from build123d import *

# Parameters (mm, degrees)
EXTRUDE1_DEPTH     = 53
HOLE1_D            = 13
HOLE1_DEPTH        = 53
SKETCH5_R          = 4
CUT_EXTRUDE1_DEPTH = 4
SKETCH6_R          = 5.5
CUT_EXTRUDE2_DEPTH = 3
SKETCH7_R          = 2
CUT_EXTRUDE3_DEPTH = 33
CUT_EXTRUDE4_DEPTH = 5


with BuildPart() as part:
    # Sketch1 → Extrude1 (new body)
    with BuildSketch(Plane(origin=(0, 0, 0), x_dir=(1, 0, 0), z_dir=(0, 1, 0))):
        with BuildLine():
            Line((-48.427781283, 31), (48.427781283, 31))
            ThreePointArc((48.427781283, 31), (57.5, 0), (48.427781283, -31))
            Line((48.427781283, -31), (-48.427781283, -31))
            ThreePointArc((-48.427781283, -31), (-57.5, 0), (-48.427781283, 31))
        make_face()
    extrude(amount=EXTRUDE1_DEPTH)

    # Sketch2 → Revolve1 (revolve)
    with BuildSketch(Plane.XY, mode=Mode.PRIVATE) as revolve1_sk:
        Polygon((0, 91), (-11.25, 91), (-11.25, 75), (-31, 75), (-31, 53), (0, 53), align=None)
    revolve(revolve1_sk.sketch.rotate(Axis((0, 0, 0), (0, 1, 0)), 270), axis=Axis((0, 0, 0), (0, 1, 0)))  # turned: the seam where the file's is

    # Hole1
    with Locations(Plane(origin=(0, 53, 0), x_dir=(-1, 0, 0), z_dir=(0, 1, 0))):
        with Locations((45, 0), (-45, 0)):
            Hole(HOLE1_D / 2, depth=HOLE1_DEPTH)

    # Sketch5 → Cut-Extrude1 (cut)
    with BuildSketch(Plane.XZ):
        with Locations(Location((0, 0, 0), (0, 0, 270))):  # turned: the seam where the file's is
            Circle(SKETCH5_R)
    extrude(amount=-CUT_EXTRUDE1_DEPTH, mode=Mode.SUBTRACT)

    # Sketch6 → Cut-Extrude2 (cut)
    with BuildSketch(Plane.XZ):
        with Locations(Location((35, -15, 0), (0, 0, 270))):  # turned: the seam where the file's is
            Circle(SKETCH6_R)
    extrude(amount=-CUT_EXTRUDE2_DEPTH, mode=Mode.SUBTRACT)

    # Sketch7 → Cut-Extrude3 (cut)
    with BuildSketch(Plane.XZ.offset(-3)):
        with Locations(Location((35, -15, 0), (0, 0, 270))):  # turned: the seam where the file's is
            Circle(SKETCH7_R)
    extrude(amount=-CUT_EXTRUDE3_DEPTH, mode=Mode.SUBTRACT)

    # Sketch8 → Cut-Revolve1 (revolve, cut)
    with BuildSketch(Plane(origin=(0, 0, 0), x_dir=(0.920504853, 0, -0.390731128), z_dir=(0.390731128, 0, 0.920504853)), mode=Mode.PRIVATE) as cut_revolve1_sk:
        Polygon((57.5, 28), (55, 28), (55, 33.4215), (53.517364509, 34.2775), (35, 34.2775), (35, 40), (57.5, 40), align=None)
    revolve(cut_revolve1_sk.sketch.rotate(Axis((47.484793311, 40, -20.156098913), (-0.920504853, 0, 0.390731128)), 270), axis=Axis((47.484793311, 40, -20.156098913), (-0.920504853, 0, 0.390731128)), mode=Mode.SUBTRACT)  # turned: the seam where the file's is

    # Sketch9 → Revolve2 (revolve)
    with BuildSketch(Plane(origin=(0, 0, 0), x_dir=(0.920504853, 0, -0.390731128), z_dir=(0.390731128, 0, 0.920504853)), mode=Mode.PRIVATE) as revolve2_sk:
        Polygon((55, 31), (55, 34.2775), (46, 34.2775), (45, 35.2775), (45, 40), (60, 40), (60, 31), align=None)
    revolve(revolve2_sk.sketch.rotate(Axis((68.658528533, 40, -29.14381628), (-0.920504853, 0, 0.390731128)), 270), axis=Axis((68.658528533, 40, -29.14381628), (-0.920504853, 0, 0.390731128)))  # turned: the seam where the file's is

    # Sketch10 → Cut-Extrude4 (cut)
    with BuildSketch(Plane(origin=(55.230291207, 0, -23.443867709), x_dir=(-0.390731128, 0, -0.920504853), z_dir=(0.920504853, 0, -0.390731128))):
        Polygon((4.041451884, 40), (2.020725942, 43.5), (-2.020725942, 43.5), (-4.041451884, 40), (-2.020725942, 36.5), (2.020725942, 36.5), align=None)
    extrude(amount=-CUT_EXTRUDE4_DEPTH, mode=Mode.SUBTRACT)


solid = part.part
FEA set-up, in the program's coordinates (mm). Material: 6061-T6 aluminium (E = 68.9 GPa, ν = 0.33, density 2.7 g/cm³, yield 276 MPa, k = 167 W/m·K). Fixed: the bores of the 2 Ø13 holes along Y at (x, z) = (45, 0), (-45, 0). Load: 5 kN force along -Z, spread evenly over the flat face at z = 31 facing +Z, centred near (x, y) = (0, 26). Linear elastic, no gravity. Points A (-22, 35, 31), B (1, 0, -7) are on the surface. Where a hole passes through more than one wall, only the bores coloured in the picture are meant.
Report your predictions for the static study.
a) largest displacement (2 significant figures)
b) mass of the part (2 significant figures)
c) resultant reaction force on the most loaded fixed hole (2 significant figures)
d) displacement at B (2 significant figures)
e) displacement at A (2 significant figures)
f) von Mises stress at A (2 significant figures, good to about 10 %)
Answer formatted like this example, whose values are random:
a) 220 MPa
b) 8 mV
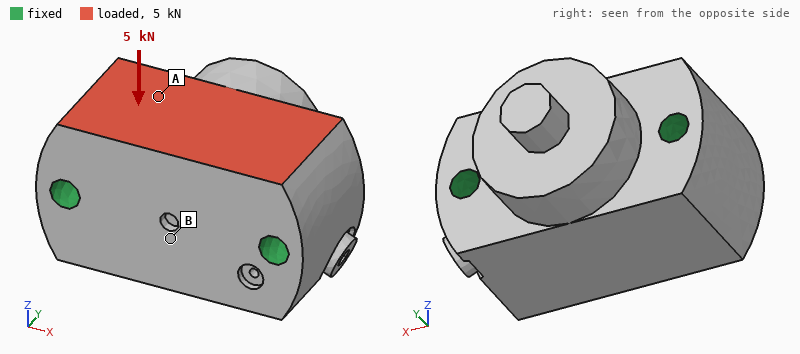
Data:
a) 1.4 µm
b) 1.1 kg
c) 2.5 kN
d) 0.99 µm
e) 0.98 µm
f) 0.91 MPa
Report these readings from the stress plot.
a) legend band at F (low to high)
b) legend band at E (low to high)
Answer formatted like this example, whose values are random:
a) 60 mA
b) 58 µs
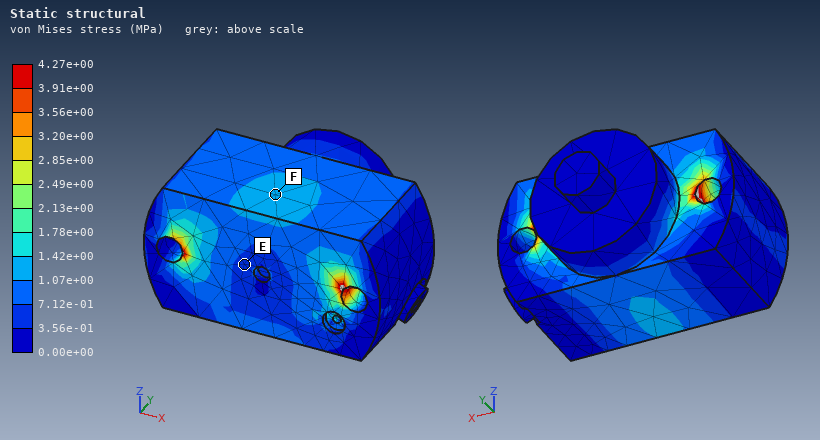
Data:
a) 1.07e+00 to 1.42e+00 MPa
b) 3.56e-01 to 7.12e-01 MPa
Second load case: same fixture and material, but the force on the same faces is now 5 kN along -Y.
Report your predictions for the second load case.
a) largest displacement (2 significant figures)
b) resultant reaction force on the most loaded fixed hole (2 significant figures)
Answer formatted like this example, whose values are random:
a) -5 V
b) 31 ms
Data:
a) 4.1 µm
b) 2.5 kN
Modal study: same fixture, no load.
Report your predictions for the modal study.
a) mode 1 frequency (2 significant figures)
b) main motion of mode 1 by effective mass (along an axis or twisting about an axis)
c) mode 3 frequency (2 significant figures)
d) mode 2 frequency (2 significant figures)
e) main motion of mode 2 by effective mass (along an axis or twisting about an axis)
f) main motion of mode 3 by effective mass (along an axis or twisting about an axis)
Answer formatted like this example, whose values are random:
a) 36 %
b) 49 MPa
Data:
a) 8200 Hz
b) along Z
c) 13 kHz
d) 12 kHz
e) along Y
f) along Z
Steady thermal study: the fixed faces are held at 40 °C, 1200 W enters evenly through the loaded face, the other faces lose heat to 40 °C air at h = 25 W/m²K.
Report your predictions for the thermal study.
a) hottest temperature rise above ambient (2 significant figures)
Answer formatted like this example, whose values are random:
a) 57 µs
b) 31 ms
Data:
a) 57 K
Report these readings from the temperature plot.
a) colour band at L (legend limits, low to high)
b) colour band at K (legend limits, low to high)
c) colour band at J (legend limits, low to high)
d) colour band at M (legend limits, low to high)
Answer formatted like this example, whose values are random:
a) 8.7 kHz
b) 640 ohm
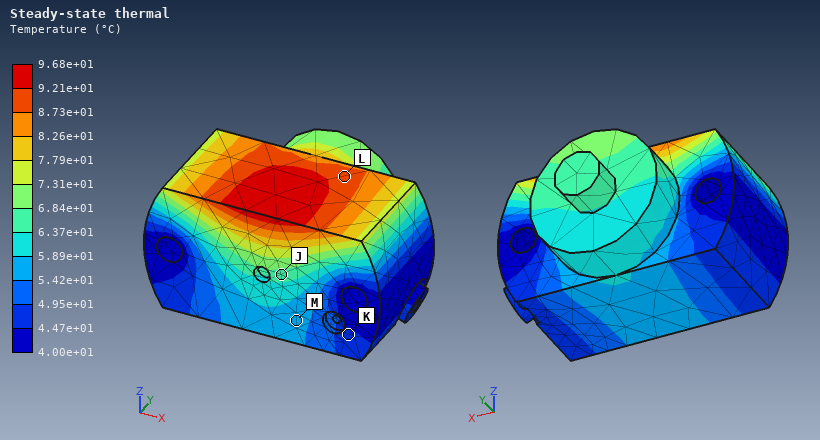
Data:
a) 8.73e+01 to 9.21e+01 °C
b) 4.47e+01 to 4.95e+01 °C
c) 6.37e+01 to 6.84e+01 °C
d) 5.42e+01 to 5.89e+01 °C
